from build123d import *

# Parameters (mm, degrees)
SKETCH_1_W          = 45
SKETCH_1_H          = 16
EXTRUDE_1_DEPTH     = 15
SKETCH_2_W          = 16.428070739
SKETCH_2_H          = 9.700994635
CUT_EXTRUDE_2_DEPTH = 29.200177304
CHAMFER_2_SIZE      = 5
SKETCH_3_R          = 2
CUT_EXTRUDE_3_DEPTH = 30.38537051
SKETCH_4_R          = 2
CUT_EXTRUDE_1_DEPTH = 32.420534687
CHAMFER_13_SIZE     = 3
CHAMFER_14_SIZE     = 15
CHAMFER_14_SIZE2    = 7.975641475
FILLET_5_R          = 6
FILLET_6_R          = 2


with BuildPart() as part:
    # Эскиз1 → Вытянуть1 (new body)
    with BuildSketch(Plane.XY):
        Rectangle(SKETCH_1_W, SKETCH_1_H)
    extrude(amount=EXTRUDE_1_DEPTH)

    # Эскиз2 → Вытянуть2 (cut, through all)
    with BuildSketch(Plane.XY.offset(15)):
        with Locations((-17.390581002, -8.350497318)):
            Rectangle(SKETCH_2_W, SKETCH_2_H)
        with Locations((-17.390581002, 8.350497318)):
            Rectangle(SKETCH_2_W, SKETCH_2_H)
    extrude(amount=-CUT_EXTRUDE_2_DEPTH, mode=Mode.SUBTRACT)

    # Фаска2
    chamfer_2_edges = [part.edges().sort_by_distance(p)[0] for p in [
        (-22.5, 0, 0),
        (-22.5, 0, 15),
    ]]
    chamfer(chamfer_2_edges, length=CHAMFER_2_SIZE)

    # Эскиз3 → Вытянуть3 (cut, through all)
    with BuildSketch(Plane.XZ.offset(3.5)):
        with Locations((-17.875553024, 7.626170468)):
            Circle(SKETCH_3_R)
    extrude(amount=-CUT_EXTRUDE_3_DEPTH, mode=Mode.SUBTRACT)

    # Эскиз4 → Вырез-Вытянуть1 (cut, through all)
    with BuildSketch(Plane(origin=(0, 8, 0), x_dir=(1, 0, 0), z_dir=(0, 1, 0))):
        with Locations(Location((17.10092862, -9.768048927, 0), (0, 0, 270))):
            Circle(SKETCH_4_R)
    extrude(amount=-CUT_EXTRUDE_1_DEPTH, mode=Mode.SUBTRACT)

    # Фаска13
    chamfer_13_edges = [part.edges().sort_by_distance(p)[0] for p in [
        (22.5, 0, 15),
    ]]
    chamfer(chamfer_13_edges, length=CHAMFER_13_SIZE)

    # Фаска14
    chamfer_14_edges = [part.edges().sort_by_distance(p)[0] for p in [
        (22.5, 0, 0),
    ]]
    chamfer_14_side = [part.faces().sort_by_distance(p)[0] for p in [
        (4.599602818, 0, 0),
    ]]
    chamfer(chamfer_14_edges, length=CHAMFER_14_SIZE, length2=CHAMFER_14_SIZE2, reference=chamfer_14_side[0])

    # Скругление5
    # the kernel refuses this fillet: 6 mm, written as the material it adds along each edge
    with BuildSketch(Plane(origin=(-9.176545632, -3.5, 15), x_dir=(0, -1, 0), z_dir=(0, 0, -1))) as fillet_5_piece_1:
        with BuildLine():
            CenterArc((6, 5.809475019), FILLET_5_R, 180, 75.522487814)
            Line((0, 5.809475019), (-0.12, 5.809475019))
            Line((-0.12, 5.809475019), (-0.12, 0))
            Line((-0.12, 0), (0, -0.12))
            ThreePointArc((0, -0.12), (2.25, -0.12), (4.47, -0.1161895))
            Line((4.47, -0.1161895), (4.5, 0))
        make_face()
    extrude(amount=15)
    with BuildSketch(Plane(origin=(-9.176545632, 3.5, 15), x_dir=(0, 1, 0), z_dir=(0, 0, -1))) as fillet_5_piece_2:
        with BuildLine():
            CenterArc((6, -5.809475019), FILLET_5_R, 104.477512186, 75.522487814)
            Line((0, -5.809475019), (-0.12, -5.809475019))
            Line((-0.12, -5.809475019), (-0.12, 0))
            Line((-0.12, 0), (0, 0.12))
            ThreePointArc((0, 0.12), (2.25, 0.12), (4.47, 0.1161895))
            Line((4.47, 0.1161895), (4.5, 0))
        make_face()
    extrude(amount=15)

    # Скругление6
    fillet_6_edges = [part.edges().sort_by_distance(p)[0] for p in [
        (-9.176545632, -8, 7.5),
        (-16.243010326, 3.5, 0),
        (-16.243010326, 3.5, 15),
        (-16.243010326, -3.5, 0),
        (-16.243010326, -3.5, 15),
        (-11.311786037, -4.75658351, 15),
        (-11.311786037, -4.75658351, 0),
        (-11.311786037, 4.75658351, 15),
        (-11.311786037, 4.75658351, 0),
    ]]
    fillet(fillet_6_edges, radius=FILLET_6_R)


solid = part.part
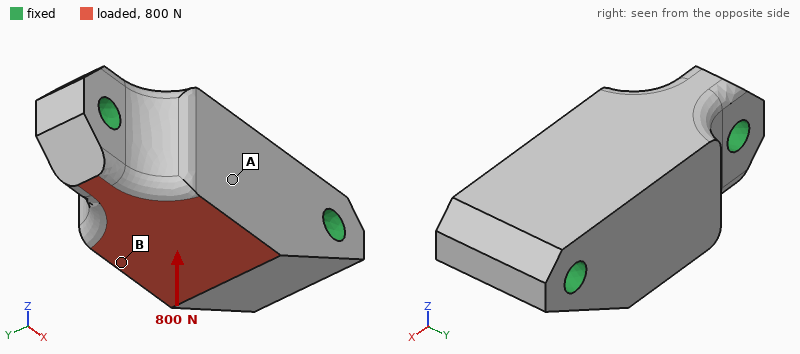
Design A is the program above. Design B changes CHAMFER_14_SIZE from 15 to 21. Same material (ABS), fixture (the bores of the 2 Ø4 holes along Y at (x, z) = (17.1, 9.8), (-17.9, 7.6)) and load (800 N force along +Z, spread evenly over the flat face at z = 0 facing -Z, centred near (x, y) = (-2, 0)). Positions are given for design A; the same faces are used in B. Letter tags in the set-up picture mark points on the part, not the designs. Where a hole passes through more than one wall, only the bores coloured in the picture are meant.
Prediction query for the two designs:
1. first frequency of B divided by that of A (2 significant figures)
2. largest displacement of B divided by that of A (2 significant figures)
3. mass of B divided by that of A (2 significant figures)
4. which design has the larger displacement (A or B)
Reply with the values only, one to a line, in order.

0.99
1.1
0.95
B
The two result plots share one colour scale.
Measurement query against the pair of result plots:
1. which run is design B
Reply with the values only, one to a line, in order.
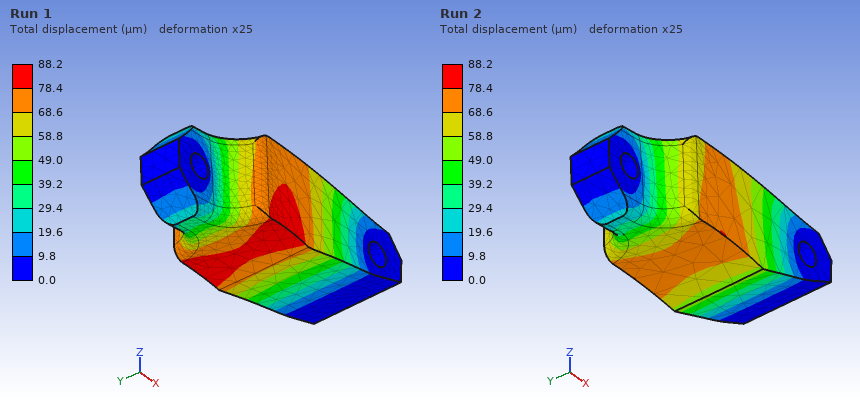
Run 1
